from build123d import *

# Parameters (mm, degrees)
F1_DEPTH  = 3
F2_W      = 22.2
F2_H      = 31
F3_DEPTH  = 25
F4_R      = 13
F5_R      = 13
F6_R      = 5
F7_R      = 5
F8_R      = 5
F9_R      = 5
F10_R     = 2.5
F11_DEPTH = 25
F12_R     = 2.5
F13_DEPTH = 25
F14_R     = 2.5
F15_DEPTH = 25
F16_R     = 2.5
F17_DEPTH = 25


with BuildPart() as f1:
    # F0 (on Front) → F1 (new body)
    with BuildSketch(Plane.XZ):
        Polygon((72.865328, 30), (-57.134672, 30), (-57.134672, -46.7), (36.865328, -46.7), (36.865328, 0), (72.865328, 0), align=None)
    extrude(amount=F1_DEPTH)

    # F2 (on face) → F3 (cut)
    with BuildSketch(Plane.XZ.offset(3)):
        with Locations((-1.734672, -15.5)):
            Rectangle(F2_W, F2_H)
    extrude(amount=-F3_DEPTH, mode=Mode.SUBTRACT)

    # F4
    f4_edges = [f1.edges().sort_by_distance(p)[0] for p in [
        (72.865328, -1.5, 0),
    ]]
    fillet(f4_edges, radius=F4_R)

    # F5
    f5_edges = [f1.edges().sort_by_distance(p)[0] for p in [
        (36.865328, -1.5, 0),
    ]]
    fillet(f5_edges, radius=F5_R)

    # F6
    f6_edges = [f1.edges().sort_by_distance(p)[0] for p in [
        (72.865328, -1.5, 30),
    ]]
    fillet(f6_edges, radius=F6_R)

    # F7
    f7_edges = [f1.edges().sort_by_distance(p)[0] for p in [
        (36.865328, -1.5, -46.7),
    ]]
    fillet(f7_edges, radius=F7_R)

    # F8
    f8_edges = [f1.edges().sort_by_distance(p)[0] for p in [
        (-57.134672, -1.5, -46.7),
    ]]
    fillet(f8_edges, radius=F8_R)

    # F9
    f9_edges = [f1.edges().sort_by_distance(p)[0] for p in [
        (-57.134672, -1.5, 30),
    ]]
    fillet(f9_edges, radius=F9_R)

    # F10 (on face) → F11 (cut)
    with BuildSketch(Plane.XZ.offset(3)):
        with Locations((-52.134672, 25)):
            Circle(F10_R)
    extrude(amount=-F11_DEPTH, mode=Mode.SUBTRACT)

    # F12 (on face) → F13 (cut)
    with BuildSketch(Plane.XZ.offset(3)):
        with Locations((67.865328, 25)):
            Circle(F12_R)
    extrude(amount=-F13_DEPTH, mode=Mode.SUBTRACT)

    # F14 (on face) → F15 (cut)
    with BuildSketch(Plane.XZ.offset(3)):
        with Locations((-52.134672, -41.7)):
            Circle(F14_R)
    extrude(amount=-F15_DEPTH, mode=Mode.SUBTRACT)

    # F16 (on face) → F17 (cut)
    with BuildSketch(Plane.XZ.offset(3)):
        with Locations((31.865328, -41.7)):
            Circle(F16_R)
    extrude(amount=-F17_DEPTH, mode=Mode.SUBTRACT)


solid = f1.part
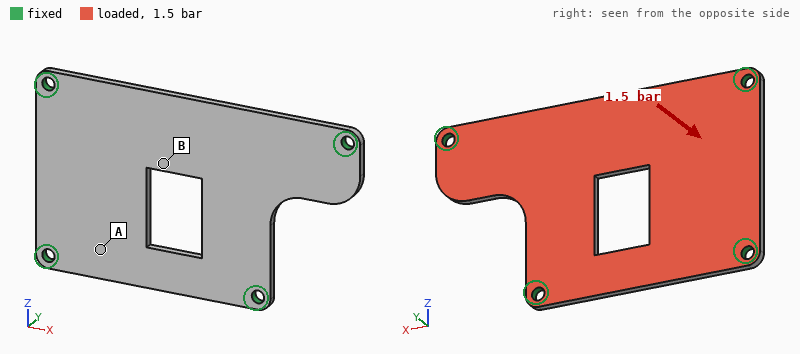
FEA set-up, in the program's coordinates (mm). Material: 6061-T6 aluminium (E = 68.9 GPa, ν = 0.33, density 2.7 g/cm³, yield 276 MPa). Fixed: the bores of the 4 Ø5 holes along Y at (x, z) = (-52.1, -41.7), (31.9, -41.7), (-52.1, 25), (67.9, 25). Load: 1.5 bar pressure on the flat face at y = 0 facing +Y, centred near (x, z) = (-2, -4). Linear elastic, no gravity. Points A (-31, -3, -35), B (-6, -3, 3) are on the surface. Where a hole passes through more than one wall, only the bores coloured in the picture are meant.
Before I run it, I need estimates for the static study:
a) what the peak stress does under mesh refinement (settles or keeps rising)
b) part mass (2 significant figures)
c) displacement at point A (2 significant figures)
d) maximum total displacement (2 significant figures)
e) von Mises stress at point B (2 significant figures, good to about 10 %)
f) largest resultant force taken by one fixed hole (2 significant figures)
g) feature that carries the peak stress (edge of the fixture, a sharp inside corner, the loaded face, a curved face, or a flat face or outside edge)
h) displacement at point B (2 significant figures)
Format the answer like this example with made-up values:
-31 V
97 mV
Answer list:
keeps rising
61 g
0.13 mm
0.57 mm
55 MPa
330 N
edge of the fixture
0.46 mm
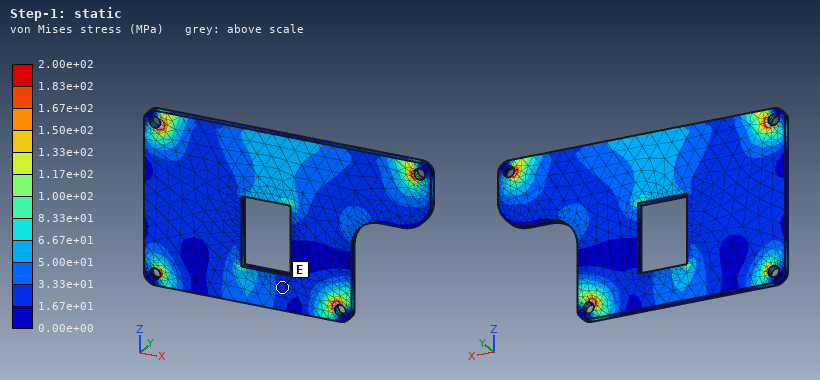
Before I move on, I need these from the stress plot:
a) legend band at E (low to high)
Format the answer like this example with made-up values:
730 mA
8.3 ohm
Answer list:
1.67e+01 to 3.33e+01 MPa
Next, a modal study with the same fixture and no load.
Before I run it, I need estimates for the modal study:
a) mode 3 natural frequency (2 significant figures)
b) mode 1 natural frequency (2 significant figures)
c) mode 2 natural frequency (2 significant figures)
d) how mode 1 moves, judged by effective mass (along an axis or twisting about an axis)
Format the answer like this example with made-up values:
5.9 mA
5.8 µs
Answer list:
2800 Hz
1200 Hz
2200 Hz
along Y
